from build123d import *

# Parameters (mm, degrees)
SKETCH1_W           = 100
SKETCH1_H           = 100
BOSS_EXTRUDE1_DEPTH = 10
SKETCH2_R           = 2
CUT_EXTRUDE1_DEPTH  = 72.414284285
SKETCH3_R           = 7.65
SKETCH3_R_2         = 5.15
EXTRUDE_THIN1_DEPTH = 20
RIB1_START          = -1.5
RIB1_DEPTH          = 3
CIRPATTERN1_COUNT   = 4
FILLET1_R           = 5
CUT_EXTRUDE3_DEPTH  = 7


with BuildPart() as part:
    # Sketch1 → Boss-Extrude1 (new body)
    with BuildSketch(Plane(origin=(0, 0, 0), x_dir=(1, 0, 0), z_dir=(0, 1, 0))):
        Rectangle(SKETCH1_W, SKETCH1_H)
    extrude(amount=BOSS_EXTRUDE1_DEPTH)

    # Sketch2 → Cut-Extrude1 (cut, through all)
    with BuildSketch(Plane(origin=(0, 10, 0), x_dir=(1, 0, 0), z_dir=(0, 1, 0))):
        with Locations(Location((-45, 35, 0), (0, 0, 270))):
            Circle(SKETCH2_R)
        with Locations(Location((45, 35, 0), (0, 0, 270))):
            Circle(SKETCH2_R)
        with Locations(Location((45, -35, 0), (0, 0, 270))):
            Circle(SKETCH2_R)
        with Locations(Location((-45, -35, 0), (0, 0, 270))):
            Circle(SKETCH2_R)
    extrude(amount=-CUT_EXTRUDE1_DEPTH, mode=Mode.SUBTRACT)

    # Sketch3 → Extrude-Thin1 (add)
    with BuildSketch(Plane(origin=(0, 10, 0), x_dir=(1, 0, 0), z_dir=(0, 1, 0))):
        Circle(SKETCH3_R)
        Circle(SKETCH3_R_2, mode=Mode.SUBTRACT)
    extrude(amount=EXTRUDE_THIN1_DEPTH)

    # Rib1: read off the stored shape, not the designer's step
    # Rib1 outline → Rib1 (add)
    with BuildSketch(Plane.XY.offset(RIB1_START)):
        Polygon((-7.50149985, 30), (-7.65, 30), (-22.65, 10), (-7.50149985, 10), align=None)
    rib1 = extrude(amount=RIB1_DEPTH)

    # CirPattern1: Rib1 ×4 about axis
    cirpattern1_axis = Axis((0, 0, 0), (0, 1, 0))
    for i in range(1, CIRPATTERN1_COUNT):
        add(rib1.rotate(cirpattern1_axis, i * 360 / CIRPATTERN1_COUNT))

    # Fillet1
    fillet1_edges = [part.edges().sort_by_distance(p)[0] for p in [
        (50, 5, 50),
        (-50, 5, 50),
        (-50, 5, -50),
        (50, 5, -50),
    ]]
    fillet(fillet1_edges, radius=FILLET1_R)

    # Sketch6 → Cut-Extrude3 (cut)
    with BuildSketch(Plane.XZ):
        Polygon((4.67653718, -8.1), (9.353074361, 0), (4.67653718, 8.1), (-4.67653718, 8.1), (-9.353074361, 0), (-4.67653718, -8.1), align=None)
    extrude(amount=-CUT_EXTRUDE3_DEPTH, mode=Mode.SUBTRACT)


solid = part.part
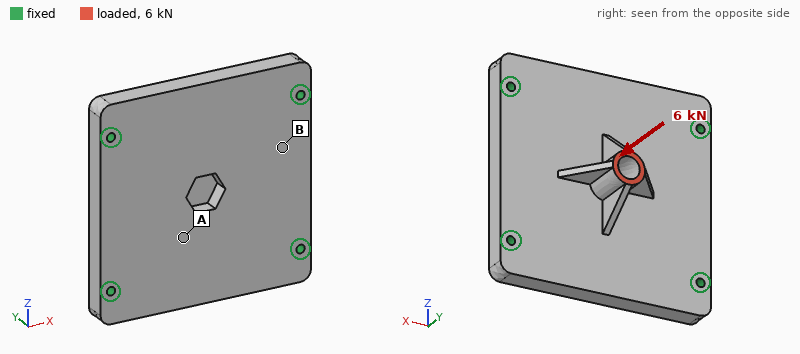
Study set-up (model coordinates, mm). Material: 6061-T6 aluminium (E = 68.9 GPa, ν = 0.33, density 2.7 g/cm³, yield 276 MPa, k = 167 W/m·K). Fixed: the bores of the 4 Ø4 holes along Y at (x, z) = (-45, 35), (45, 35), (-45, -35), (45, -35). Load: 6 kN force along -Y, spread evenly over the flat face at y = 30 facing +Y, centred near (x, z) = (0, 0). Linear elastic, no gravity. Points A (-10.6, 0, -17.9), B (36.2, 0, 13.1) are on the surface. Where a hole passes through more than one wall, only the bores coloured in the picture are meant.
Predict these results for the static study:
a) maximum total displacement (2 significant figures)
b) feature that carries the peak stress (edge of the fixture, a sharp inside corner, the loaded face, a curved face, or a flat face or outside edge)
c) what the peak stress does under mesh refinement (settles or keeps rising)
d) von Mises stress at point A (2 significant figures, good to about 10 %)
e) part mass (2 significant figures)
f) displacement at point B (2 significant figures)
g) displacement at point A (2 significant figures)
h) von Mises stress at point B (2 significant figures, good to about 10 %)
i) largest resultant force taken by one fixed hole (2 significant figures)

97 µm
edge of the fixture
keeps rising
31 MPa
270 g
34 µm
72 µm
16 MPa
1.5 kN
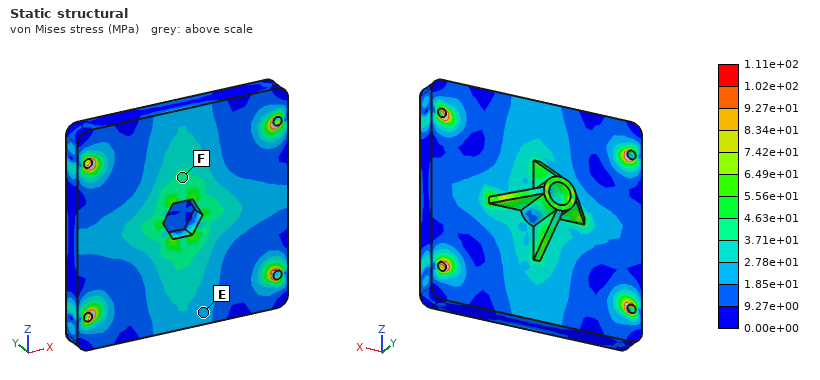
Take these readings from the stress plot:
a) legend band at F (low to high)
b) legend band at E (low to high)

3.71e+01 to 4.63e+01 MPa
1.85e+01 to 2.78e+01 MPa
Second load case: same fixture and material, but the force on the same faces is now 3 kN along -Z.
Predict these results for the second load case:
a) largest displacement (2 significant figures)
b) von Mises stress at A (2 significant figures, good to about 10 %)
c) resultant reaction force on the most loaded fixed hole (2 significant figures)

75 µm
13 MPa
980 N
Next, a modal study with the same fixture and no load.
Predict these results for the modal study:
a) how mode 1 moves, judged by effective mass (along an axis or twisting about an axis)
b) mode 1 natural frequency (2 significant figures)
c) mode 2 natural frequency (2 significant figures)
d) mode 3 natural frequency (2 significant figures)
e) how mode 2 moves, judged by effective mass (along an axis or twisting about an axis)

along Y
4200 Hz
5800 Hz
7700 Hz
twisting about X
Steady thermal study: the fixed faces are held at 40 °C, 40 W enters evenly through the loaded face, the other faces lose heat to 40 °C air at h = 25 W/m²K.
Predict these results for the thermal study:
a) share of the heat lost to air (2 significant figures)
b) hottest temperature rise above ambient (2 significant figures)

9.5 %
40 K
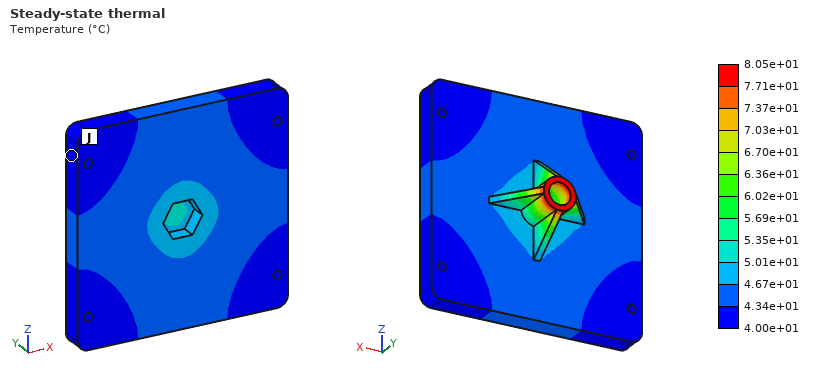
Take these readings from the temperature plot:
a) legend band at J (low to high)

4.00e+01 to 4.34e+01 °C
